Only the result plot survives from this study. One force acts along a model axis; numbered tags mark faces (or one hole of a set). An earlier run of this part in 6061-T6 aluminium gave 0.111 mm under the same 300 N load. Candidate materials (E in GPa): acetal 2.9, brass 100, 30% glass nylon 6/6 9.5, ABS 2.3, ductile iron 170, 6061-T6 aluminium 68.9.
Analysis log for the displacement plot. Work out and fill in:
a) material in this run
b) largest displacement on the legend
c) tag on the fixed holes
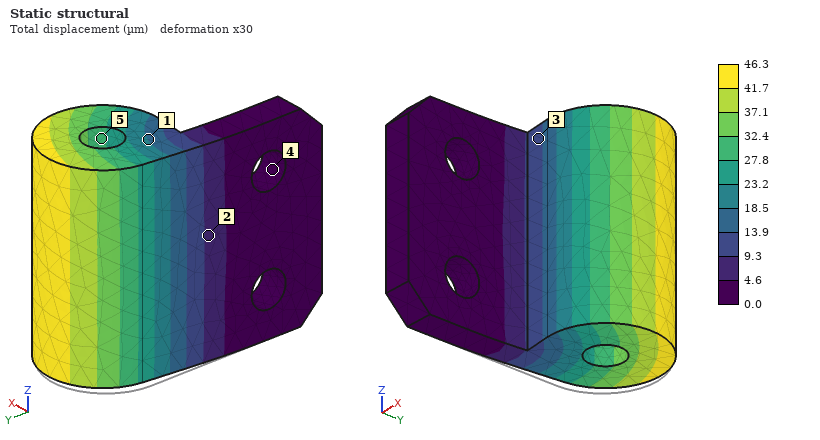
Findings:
ductile iron
46.3 µm
4
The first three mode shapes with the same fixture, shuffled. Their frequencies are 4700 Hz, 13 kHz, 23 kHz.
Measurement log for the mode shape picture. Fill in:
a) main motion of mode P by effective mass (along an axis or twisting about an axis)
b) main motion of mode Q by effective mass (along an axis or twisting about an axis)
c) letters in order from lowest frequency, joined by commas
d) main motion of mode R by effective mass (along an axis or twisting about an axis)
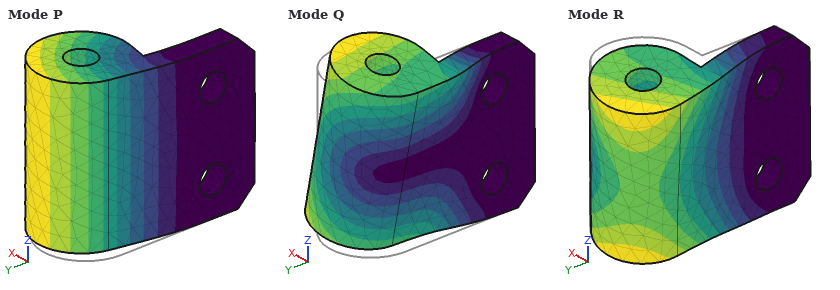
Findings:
along X
along Z
P, Q, R
along Z
